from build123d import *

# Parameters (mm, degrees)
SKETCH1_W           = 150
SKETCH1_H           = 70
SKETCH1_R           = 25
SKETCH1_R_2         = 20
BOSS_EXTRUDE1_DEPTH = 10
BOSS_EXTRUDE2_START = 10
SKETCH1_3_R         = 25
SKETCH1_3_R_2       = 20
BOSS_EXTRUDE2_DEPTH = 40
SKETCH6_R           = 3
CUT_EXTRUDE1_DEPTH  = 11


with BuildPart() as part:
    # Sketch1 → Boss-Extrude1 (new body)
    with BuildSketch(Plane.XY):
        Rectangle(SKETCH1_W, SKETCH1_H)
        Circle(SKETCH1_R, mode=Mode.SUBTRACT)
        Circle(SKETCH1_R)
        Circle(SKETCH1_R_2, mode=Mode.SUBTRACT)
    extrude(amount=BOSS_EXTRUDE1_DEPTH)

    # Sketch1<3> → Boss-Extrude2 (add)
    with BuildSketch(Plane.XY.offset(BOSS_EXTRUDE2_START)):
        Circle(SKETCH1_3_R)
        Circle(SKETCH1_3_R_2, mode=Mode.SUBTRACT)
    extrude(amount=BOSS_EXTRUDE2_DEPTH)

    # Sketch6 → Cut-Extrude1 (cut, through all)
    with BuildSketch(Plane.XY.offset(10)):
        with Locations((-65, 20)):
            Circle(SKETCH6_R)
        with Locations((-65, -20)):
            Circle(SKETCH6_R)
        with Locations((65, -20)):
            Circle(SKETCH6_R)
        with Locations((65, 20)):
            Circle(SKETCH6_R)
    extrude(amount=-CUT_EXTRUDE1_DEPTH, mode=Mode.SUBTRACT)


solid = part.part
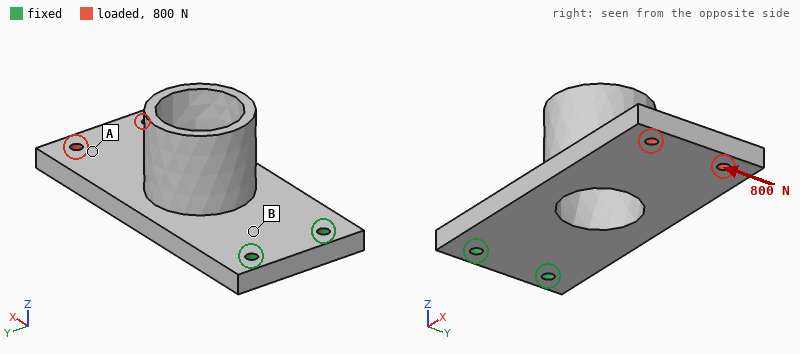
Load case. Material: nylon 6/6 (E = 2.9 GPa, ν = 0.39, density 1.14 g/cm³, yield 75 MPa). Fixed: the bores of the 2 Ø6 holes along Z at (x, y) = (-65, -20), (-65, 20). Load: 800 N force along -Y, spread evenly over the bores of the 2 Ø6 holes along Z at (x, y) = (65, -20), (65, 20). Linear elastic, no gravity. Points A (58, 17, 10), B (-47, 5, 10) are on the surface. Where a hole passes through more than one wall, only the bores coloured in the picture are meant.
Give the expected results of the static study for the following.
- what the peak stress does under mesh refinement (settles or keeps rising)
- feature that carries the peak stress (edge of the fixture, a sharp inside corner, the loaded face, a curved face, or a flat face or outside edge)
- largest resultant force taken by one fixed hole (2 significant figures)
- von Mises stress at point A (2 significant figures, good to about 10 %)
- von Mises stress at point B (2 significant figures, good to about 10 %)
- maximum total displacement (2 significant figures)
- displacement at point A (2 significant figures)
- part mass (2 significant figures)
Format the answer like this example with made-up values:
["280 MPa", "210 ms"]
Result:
["keeps rising", "edge of the fixture", "2.4 kN", "2.6 MPa", "5.4 MPa", "1.5 mm", "1.2 mm", "140 g"]
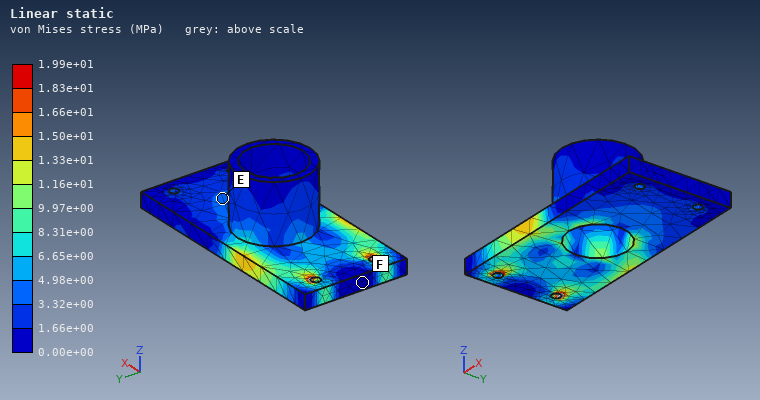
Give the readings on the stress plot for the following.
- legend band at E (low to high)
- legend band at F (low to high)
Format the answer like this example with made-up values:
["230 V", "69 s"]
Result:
["3.32e+00 to 4.98e+00 MPa", "0.00e+00 to 1.66e+00 MPa"]
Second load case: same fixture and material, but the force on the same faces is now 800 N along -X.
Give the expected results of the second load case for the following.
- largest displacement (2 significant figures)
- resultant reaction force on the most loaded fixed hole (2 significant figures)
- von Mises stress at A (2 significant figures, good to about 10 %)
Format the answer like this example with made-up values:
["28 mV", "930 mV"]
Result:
["0.16 mm", "400 N", "1.8 MPa"]
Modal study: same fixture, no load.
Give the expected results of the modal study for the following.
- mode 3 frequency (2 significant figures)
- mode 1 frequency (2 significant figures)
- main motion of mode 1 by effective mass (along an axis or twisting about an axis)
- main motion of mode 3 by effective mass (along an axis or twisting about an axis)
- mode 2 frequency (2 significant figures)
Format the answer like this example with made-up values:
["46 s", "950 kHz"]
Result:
["590 Hz", "130 Hz", "along Z", "along Y", "460 Hz"]
